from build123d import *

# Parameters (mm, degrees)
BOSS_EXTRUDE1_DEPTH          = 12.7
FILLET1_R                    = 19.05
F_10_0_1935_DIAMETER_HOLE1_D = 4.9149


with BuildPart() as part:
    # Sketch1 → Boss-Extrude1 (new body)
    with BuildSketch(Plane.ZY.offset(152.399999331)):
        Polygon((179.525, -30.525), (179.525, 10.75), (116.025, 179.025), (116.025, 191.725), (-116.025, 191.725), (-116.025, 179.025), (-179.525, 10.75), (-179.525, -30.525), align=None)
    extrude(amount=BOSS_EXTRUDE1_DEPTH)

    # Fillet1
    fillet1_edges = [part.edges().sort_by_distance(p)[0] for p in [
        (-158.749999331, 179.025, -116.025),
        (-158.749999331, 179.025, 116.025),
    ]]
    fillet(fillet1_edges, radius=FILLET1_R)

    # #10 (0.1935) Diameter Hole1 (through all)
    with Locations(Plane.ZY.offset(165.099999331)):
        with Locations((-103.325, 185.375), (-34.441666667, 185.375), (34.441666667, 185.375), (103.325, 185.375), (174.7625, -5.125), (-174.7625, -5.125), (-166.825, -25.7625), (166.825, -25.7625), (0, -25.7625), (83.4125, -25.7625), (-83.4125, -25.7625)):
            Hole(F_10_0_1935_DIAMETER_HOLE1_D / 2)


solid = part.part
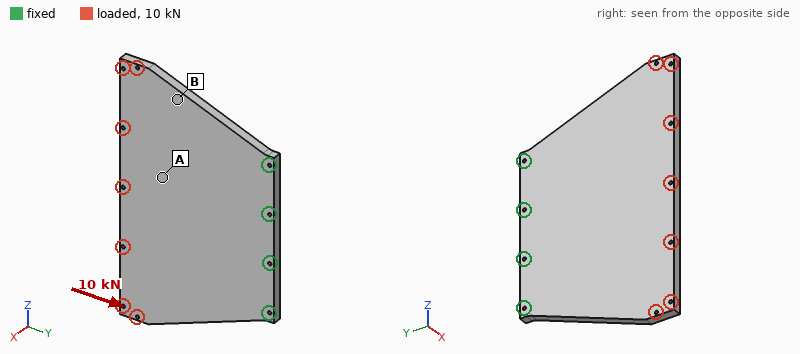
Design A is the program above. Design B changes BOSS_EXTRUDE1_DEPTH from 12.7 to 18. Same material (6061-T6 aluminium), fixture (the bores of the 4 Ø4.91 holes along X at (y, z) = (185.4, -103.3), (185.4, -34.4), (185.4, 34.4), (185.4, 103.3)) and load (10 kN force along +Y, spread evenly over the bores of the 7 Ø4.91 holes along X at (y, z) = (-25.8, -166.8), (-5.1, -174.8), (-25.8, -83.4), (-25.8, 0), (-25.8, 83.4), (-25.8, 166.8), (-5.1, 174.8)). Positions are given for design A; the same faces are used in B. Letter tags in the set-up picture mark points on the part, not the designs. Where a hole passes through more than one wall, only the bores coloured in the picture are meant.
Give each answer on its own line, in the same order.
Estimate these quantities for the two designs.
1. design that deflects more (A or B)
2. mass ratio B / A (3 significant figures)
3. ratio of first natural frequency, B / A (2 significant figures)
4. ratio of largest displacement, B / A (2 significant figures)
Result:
A
1.42
1.4
0.71
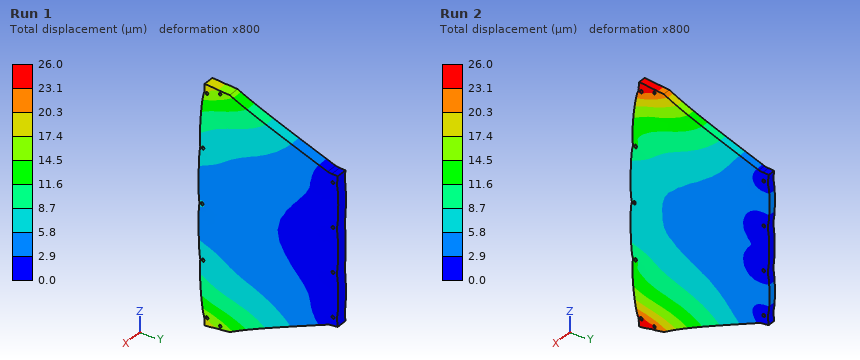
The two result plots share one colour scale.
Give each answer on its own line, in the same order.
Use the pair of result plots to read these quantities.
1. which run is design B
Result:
Run 1
